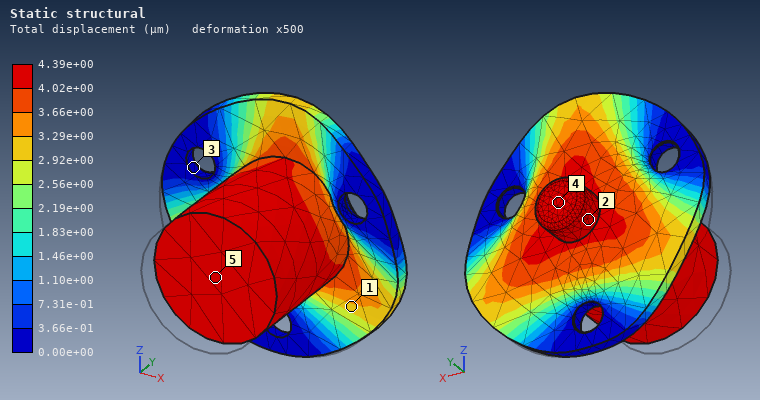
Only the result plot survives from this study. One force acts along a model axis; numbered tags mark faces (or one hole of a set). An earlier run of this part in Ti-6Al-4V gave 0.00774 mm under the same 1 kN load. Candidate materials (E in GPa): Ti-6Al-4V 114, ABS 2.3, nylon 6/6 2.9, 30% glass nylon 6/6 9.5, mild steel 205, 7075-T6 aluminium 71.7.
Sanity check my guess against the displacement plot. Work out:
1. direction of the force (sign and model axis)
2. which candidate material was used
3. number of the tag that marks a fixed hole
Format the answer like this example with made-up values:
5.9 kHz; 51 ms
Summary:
+Y; mild steel; 3
